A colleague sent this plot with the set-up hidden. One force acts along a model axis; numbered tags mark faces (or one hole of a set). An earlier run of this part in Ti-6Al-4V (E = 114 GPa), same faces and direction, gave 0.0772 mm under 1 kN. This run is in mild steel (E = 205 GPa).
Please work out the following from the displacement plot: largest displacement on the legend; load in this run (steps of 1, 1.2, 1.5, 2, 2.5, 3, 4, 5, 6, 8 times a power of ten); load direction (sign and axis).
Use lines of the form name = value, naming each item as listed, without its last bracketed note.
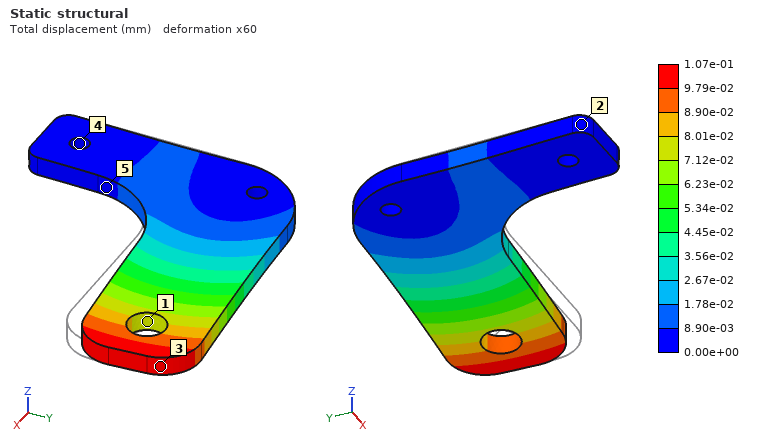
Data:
largest displacement on the legend = 1.07e-01 mm
load in this run = 2.5 kN
load direction = +Y
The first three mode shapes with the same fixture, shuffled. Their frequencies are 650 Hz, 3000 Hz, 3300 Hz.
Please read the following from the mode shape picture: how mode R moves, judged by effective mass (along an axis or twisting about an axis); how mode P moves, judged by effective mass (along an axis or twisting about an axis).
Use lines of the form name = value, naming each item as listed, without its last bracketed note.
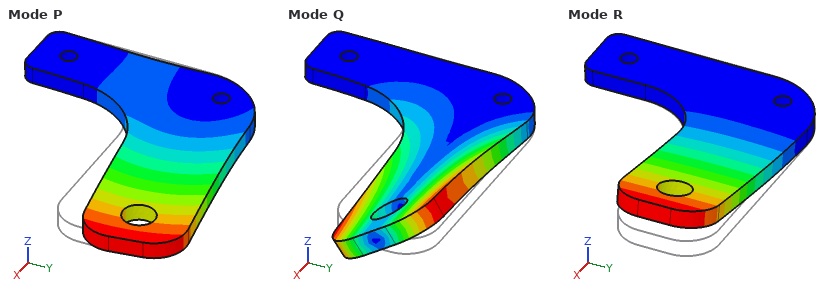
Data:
how mode R moves, judged by effective mass = along Z
how mode P moves, judged by effective mass = along Y
